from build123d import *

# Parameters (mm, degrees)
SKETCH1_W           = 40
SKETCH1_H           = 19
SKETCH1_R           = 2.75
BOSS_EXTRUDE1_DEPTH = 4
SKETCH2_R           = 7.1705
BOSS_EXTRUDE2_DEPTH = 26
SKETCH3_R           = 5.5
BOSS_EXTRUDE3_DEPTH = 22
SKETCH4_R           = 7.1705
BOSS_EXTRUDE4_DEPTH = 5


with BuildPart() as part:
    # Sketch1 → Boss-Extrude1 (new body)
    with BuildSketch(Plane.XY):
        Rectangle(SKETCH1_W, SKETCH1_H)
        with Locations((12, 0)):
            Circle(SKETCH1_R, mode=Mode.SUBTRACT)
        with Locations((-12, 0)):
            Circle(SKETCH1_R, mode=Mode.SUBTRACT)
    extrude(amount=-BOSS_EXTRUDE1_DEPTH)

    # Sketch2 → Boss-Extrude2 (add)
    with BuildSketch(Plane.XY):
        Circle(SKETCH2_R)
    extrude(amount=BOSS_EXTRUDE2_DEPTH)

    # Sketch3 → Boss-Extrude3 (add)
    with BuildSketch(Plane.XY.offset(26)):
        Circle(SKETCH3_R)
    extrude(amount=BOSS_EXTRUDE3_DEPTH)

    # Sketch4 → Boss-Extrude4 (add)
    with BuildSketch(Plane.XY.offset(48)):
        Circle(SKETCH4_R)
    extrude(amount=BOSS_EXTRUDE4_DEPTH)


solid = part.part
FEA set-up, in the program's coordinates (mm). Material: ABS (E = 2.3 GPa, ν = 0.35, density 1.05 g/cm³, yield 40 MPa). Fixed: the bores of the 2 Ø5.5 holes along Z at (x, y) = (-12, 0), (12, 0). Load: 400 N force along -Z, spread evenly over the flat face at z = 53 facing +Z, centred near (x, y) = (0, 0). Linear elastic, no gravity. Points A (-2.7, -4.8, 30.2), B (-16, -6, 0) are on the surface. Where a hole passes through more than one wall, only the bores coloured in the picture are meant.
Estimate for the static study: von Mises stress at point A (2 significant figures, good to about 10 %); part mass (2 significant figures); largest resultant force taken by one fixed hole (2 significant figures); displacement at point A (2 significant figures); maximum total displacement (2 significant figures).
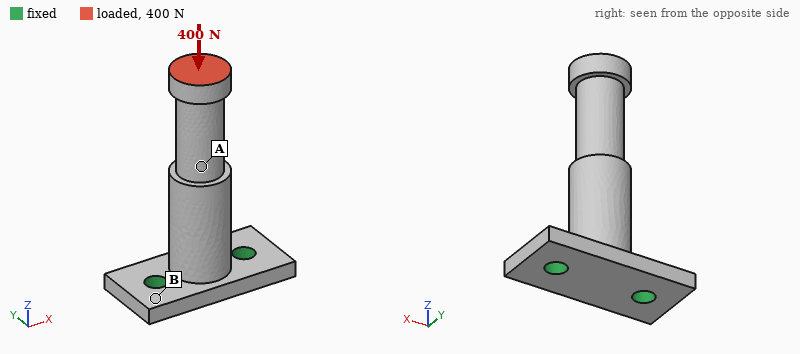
4.1 MPa
10 g
210 N
0.082 mm
0.12 mm
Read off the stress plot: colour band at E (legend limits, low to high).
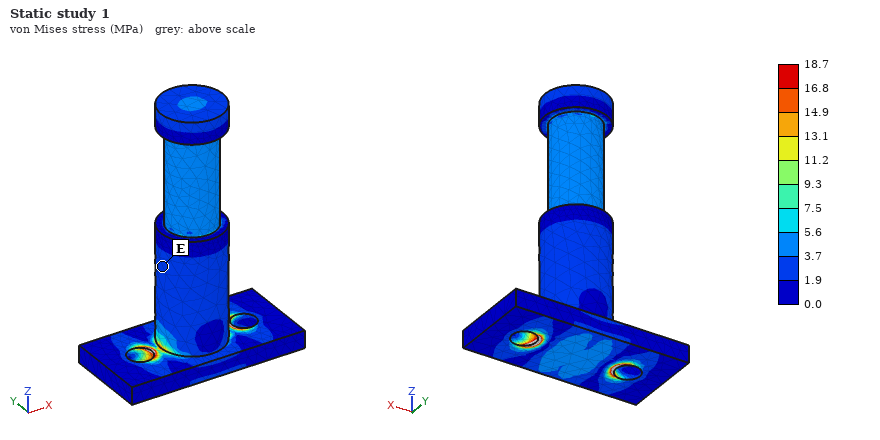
1.9 to 3.7 MPa
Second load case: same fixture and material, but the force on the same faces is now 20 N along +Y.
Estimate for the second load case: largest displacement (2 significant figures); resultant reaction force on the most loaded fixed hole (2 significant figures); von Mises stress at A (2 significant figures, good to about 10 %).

0.73 mm
10 N
3.0 MPa
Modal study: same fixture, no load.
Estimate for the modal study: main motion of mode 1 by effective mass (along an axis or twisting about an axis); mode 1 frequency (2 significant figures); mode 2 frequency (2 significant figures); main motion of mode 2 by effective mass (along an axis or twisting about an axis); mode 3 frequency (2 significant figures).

along Y
590 Hz
910 Hz
along X
3400 Hz
